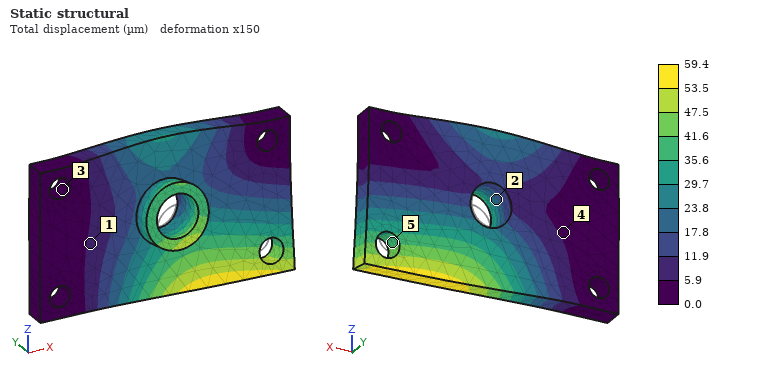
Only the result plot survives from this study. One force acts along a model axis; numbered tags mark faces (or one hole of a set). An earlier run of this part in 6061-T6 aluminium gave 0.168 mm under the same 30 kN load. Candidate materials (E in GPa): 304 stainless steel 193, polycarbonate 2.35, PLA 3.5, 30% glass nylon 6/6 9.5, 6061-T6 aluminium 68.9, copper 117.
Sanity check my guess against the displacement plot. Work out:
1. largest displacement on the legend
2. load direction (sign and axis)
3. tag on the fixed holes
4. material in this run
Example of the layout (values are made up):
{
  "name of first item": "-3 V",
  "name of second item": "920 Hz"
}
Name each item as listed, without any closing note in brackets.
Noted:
{
  "largest displacement on the legend": "59.4 µm",
  "load direction": "+Z",
  "tag on the fixed holes": "3",
  "material in this run": "304 stainless steel"
}
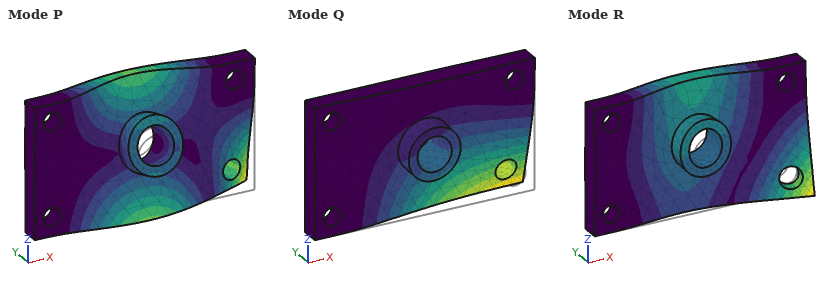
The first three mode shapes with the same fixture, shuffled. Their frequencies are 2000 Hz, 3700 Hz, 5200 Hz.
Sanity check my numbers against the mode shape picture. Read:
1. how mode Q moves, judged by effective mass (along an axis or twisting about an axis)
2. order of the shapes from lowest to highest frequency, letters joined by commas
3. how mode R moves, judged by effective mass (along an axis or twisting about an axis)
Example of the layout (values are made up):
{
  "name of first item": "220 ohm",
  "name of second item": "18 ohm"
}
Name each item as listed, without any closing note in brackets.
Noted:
{
  "how mode Q moves, judged by effective mass": "along Y",
  "order of the shapes from lowest to highest frequency, letters joined by commas": "Q, R, P",
  "how mode R moves, judged by effective mass": "along Y"
}
